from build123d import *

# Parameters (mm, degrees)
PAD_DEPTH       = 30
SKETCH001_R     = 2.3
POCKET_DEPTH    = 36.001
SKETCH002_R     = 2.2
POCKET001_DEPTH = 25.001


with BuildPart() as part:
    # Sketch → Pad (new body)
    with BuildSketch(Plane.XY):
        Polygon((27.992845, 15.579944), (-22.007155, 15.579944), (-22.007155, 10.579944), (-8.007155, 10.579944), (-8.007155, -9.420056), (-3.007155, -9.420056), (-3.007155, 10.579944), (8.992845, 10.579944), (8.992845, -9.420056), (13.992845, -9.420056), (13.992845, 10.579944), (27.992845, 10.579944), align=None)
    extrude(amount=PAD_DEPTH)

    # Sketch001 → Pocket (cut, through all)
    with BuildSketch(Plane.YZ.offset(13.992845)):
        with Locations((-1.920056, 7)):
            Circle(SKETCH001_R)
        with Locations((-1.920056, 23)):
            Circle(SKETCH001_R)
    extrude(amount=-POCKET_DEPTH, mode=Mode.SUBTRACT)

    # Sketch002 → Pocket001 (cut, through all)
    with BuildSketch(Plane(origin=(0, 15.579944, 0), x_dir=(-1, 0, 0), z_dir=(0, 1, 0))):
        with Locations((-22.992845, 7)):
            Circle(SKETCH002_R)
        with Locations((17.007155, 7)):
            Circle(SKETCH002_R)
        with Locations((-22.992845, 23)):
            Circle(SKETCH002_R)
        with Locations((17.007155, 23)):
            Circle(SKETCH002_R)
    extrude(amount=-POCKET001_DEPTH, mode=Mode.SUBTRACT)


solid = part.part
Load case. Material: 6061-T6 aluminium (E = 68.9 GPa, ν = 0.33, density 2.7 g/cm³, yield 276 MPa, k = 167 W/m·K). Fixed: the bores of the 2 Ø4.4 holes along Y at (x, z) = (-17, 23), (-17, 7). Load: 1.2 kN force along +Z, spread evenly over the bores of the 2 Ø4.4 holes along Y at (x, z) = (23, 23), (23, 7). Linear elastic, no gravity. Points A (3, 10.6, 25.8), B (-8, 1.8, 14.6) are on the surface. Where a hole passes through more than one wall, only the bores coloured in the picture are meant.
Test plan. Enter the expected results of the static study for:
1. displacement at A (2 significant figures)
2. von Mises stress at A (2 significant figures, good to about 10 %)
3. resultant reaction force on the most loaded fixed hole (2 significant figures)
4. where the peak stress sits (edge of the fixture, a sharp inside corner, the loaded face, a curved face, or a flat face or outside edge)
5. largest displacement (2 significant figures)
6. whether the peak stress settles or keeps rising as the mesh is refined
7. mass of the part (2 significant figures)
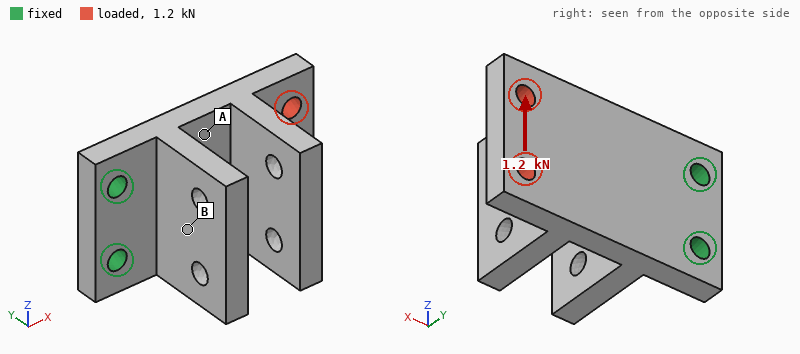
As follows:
23 µm
26 MPa
2.6 kN
edge of the fixture
65 µm
keeps rising
35 g
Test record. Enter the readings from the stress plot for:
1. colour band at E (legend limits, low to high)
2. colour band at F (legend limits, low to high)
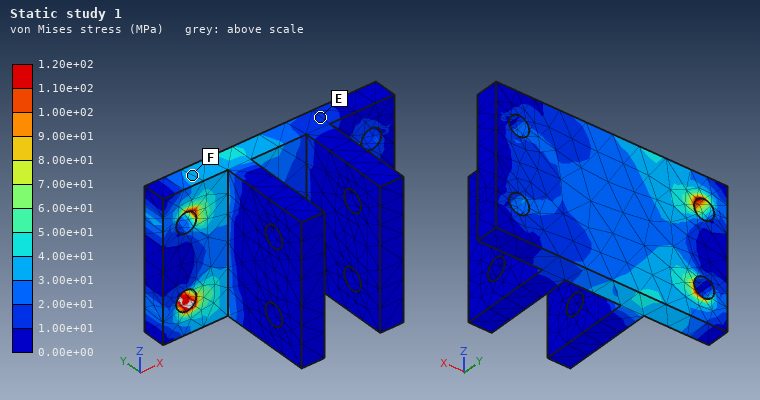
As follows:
1.00e+01 to 2.00e+01 MPa
3.00e+01 to 4.00e+01 MPa
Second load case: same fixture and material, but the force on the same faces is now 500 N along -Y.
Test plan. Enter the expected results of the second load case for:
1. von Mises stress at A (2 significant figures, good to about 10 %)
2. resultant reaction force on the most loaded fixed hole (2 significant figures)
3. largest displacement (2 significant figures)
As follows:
74 MPa
250 N
0.50 mm
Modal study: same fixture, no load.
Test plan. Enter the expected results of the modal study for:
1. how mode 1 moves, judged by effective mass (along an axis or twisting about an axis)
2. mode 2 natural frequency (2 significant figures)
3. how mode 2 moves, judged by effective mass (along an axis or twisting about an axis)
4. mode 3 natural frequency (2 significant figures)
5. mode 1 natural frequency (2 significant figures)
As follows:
along Y
4100 Hz
along Z
5700 Hz
1600 Hz
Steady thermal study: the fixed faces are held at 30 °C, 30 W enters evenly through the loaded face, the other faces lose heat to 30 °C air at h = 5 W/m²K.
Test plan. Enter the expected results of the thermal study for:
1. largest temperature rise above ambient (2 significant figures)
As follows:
49 K
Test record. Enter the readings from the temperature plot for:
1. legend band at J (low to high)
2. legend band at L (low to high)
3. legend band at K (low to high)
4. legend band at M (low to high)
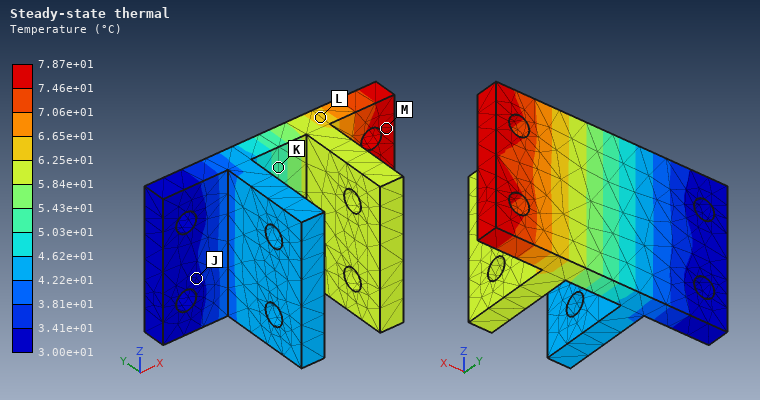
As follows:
3.00e+01 to 3.41e+01 °C
6.25e+01 to 6.65e+01 °C
5.03e+01 to 5.43e+01 °C
7.46e+01 to 7.87e+01 °C
